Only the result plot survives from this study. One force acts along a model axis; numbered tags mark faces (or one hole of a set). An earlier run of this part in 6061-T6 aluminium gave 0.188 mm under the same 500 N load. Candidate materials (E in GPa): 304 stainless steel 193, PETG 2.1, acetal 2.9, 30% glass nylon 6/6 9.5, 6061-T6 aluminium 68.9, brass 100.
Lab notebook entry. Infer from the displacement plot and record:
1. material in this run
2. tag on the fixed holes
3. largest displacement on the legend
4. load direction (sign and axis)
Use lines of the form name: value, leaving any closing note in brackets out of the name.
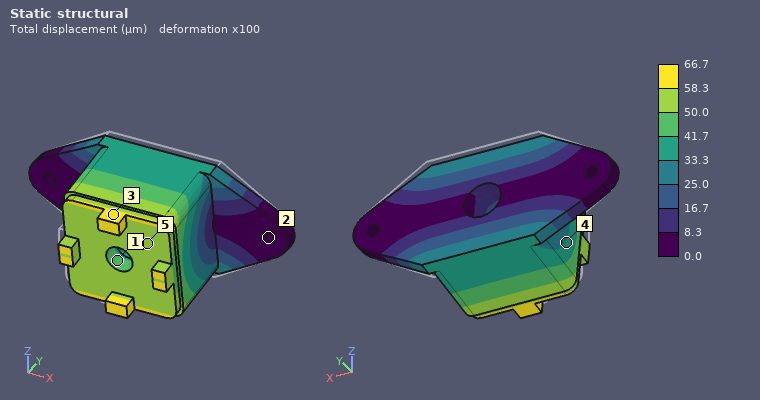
material in this run: 304 stainless steel
tag on the fixed holes: 2
largest displacement on the legend: 66.7 µm
load direction: -Z
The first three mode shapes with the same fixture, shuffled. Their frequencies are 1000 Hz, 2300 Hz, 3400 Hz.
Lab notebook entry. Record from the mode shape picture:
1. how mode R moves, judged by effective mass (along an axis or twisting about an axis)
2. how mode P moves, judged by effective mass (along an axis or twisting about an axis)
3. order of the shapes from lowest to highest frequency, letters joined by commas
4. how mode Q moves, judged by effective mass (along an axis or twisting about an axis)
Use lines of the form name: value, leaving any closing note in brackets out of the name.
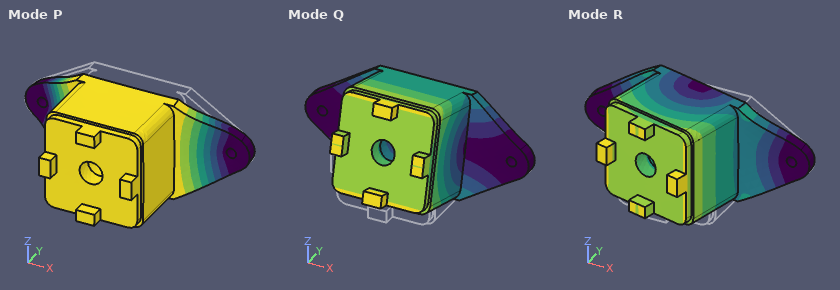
how mode R moves, judged by effective mass: along X
how mode P moves, judged by effective mass: along Y
order of the shapes from lowest to highest frequency, letters joined by commas: Q, P, R
how mode Q moves, judged by effective mass: along Z
